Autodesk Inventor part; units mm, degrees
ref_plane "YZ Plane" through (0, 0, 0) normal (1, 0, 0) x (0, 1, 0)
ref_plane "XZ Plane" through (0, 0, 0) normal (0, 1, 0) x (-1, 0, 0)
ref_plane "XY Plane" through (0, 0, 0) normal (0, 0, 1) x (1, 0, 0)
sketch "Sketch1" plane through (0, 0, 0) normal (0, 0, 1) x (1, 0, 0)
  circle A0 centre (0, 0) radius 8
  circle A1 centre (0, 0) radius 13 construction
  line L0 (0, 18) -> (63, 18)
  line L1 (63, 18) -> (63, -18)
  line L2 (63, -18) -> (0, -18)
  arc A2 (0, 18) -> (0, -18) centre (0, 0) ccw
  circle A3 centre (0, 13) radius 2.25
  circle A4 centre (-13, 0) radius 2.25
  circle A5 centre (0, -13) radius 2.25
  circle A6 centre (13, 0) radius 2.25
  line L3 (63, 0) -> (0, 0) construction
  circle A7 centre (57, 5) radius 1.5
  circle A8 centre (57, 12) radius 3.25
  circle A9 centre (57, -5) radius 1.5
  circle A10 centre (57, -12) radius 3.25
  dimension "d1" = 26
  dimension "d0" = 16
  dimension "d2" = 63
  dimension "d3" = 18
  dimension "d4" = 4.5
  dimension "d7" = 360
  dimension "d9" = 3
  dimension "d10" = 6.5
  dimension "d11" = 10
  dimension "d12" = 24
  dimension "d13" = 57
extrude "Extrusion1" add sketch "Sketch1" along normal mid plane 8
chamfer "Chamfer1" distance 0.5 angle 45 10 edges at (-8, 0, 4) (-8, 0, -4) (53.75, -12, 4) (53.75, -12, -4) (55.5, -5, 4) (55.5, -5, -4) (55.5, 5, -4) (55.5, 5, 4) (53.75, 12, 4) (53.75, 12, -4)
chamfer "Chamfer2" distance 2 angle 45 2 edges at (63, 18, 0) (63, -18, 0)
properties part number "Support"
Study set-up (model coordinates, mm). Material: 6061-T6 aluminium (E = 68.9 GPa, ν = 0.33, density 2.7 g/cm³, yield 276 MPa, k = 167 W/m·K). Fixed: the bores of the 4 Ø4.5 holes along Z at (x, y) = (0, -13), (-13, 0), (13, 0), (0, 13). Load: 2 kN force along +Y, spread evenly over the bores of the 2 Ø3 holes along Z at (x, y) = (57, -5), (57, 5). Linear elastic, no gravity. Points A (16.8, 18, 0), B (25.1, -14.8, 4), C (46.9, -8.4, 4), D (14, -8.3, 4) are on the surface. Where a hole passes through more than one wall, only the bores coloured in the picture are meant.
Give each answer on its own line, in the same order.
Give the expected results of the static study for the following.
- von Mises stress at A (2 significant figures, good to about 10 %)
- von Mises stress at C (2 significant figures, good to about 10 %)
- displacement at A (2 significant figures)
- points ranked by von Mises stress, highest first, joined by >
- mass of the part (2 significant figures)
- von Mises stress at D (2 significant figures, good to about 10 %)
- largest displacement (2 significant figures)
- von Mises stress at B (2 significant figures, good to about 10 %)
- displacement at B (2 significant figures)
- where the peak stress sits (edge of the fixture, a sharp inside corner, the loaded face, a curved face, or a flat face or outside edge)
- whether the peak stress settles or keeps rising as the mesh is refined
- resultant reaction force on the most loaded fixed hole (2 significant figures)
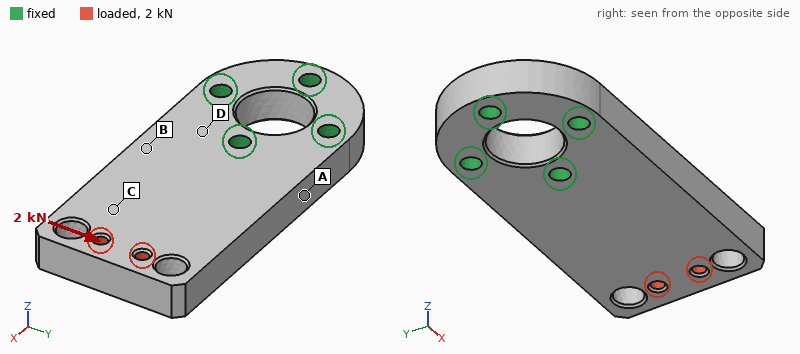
51 MPa
16 MPa
13 µm
A > B > D > C
52 g
24 MPa
76 µm
32 MPa
19 µm
edge of the fixture
keeps rising
2.8 kN
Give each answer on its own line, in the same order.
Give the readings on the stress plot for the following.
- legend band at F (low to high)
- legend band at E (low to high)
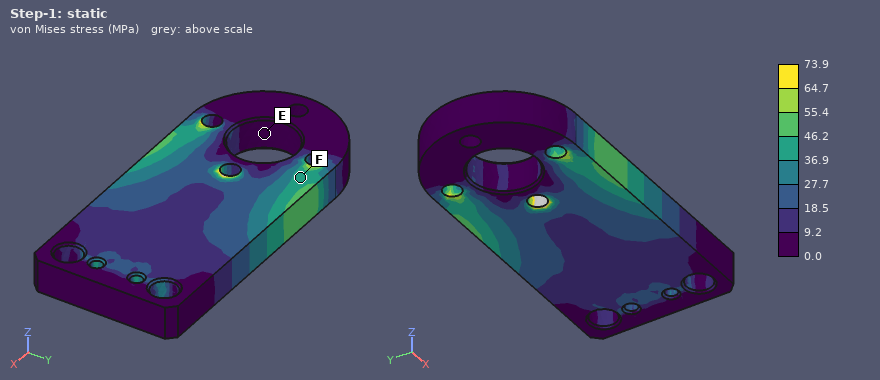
36.9 to 46.2 MPa
0.0 to 9.2 MPa
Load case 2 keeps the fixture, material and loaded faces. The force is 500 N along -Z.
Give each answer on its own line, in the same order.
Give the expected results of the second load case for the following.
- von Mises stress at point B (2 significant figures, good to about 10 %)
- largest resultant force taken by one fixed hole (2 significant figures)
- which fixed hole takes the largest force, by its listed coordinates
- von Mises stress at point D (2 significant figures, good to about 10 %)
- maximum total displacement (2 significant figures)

39 MPa
1.1 kN
(13, 0)
33 MPa
0.18 mm
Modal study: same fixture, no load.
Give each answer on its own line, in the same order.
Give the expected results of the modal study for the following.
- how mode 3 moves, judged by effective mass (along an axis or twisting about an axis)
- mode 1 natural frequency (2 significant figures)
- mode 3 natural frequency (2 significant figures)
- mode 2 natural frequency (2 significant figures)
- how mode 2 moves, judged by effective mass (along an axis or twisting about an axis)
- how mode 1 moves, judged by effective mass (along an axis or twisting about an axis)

along Y
2600 Hz
7300 Hz
6400 Hz
twisting about X
along Z
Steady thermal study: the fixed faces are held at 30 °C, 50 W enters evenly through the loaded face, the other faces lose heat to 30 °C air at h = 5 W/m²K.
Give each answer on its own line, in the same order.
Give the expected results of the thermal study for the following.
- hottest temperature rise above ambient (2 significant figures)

57 K
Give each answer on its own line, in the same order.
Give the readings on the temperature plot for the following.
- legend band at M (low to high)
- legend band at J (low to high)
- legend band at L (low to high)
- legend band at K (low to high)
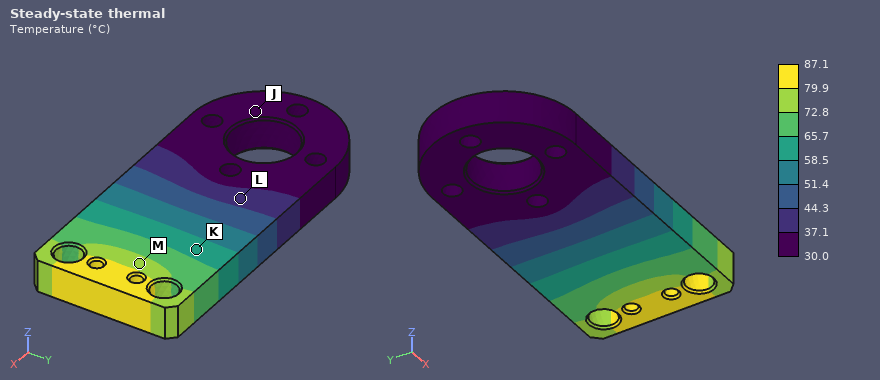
72.8 to 79.9 °C
30.0 to 37.1 °C
37.1 to 44.3 °C
58.5 to 65.7 °C
